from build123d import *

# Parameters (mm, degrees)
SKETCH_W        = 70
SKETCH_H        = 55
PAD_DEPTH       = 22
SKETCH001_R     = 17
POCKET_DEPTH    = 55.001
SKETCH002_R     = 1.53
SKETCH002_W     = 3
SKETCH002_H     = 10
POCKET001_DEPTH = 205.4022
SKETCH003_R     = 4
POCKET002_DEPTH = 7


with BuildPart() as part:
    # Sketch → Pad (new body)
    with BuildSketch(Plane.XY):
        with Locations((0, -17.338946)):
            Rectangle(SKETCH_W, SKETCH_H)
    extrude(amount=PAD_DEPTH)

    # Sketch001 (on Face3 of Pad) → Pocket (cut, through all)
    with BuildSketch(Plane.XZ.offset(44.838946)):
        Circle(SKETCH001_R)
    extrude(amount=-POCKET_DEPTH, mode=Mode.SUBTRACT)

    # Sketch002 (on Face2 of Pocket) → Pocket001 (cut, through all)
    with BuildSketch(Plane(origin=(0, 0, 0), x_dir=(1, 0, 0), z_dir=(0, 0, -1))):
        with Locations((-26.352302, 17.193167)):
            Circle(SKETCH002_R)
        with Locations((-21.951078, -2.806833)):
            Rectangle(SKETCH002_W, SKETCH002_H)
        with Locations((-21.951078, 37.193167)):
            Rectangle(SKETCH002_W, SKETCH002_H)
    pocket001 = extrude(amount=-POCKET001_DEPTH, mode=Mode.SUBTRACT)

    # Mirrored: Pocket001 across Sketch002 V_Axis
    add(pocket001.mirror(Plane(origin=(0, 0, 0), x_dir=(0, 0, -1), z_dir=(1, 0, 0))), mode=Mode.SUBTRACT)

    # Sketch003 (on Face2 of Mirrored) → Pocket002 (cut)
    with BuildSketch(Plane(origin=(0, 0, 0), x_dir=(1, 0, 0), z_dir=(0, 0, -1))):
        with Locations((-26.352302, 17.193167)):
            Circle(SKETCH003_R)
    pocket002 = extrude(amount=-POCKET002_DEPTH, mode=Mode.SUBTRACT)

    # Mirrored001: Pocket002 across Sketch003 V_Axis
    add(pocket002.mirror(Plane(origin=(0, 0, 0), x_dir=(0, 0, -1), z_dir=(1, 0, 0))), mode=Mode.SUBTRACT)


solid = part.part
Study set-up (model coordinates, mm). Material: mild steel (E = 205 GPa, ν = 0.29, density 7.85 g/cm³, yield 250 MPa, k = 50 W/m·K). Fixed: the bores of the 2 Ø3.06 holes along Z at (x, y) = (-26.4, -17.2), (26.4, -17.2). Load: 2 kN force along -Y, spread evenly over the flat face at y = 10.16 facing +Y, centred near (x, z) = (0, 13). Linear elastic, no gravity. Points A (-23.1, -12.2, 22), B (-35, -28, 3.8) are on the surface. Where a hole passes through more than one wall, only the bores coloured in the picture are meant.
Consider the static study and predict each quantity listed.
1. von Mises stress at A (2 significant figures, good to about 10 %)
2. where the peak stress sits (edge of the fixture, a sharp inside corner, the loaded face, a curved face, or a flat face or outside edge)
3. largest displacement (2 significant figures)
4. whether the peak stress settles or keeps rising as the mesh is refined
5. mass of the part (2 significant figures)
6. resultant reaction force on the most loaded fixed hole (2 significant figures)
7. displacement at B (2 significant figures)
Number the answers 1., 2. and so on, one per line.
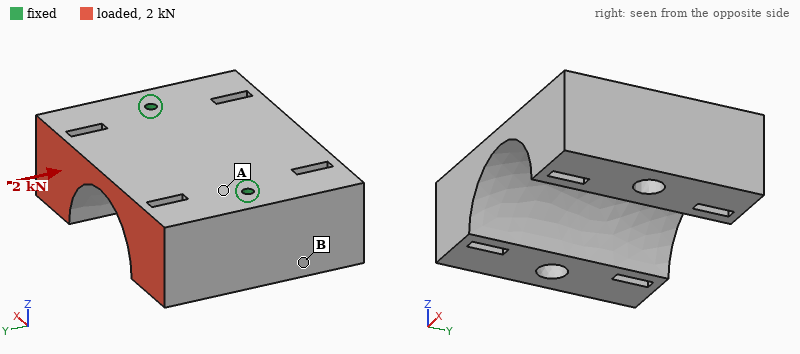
1. 3.0 MPa
2. edge of the fixture
3. 0.76 µm
4. keeps rising
5. 440 g
6. 1.0 kN
7. 0.23 µm
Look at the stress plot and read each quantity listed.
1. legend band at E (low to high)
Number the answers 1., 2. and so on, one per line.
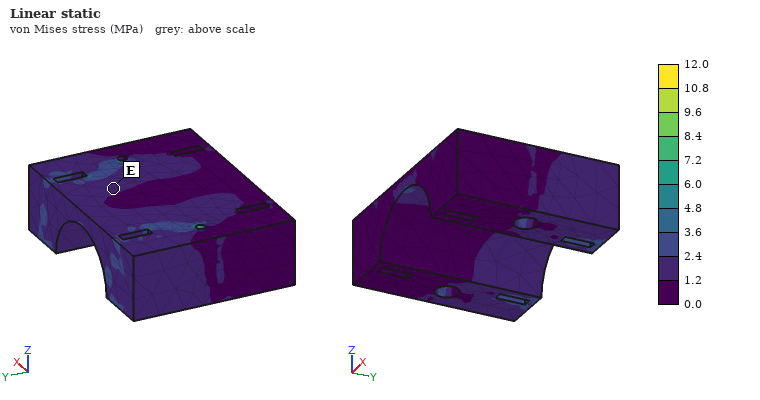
1. 1.2 to 2.4 MPa
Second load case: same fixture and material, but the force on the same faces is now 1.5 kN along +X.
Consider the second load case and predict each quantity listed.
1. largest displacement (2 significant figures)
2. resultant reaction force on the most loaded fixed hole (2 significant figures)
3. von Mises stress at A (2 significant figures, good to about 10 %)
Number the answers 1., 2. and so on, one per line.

1. 2.3 µm
2. 1.1 kN
3. 5.8 MPa
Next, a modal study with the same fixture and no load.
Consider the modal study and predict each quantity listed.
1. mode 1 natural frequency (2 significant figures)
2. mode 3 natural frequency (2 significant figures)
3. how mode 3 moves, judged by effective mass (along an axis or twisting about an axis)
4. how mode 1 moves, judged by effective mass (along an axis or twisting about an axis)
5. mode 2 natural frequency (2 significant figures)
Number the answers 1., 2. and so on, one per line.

1. 7600 Hz
2. 11 kHz
3. along Z
4. twisting about X
5. 9500 Hz
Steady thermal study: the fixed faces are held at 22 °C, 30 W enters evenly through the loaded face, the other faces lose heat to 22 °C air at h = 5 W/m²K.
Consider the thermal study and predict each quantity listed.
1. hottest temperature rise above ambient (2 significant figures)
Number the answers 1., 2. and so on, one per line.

1. 21 K
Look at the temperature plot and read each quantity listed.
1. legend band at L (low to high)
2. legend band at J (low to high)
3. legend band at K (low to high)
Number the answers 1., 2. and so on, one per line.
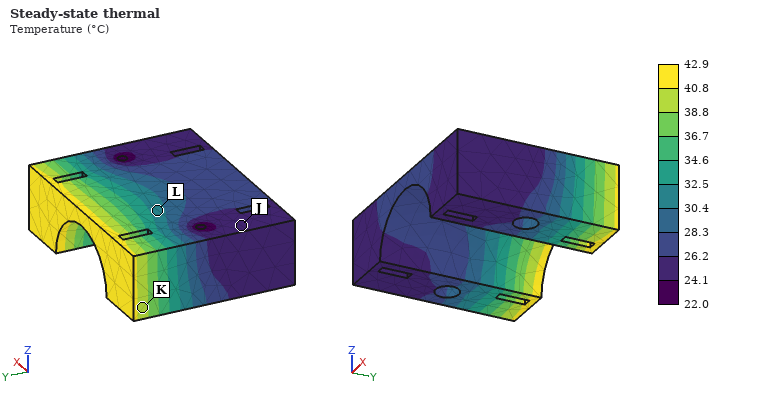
1. 30.4 to 32.5 °C
2. 24.1 to 26.2 °C
3. 38.8 to 40.8 °C
